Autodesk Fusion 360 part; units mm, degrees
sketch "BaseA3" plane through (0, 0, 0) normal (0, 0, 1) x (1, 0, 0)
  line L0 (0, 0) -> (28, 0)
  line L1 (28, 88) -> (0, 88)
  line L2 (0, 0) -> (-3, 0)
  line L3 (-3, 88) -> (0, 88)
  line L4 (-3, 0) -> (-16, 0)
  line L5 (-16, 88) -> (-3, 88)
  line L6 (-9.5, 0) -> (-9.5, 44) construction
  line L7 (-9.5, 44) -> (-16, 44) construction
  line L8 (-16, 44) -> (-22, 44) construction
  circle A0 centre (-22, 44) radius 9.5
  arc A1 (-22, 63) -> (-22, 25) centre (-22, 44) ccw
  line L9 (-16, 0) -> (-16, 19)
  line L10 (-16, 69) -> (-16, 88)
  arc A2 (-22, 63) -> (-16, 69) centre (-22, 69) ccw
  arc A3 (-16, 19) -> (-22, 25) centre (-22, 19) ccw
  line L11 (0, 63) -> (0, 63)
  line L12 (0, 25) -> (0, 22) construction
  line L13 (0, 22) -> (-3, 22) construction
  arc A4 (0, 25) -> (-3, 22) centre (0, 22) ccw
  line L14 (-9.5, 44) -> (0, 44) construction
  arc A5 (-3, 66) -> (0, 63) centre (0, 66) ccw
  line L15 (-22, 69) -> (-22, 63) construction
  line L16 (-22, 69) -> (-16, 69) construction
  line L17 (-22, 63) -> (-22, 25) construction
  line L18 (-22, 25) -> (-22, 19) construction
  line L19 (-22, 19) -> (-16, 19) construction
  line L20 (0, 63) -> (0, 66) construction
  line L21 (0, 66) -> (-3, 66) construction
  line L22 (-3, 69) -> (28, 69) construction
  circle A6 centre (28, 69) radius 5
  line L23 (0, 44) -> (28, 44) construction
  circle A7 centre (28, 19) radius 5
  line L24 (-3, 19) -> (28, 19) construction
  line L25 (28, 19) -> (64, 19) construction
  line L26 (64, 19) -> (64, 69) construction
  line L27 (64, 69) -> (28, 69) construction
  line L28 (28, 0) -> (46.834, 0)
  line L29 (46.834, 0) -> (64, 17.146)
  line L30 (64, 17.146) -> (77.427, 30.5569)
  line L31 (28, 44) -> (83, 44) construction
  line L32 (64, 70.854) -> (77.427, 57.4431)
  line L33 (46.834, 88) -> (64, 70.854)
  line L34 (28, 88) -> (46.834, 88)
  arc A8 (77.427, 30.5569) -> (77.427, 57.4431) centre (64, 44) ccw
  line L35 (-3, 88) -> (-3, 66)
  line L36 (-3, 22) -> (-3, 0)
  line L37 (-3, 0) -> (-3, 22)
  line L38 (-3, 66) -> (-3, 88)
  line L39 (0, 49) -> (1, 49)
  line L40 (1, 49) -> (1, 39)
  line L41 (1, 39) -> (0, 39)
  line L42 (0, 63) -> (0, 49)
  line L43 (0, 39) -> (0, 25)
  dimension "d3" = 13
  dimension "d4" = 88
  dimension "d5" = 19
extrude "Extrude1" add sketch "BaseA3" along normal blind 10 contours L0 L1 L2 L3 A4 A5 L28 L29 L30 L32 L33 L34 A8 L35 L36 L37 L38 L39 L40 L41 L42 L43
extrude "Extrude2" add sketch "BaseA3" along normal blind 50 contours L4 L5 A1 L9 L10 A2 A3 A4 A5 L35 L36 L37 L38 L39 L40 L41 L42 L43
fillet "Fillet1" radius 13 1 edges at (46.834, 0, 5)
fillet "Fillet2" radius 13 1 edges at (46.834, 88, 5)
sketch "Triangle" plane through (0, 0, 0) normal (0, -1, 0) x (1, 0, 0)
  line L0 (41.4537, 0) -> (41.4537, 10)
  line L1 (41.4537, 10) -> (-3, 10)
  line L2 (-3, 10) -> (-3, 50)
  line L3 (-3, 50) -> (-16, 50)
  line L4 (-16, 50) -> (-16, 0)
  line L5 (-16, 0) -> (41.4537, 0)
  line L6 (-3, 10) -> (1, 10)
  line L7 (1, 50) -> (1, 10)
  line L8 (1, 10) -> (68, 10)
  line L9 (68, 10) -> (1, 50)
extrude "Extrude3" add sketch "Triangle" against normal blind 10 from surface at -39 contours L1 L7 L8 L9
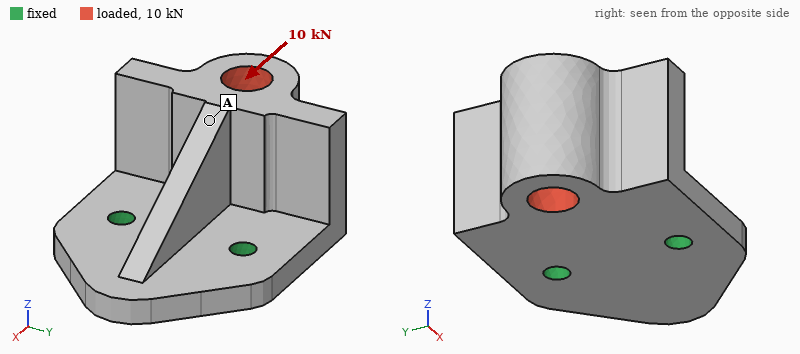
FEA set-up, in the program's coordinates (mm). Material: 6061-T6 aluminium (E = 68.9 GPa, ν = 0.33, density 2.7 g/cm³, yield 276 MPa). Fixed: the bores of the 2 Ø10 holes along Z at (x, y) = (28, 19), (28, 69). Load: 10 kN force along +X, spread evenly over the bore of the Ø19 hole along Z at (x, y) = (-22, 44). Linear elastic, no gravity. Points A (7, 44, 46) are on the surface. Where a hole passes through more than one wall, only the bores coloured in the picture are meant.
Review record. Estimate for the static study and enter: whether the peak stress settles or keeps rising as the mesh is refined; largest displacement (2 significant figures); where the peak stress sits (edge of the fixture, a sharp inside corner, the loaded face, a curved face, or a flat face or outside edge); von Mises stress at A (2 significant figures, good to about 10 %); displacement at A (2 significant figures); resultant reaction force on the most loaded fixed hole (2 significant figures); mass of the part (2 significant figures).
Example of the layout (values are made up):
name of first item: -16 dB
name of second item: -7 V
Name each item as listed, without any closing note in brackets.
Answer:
whether the peak stress settles or keeps rising as the mesh is refined: keeps rising
largest displacement: 0.28 mm
where the peak stress sits: edge of the fixture
von Mises stress at A: 21 MPa
displacement at A: 0.16 mm
resultant reaction force on the most loaded fixed hole: 5.0 kN
mass of the part: 440 g
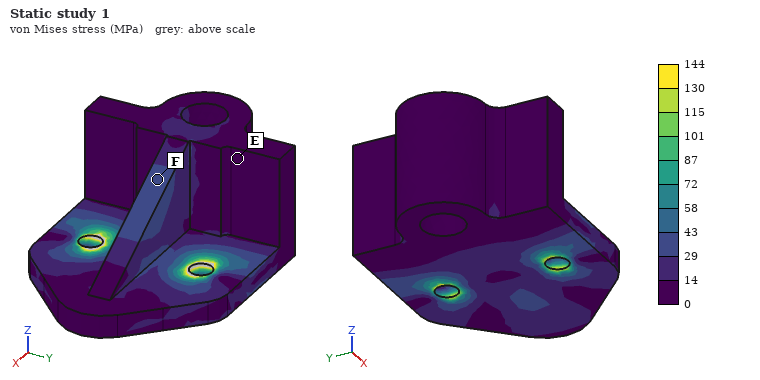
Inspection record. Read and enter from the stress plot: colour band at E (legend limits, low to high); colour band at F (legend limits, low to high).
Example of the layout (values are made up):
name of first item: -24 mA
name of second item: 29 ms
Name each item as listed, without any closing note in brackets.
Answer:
colour band at E: 0 to 14 MPa
colour band at F: 29 to 43 MPa
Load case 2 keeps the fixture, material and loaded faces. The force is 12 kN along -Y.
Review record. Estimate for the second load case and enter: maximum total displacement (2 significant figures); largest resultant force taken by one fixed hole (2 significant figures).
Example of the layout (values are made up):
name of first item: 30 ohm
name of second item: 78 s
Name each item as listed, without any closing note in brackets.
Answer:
maximum total displacement: 0.17 mm
largest resultant force taken by one fixed hole: 13 kN
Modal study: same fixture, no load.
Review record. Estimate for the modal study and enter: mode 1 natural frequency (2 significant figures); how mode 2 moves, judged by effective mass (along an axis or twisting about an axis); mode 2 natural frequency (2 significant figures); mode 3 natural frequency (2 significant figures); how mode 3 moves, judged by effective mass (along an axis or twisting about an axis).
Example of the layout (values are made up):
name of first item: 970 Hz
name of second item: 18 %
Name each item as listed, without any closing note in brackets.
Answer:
mode 1 natural frequency: 1600 Hz
how mode 2 moves, judged by effective mass: along Y
mode 2 natural frequency: 2800 Hz
mode 3 natural frequency: 5400 Hz
how mode 3 moves, judged by effective mass: along Z
